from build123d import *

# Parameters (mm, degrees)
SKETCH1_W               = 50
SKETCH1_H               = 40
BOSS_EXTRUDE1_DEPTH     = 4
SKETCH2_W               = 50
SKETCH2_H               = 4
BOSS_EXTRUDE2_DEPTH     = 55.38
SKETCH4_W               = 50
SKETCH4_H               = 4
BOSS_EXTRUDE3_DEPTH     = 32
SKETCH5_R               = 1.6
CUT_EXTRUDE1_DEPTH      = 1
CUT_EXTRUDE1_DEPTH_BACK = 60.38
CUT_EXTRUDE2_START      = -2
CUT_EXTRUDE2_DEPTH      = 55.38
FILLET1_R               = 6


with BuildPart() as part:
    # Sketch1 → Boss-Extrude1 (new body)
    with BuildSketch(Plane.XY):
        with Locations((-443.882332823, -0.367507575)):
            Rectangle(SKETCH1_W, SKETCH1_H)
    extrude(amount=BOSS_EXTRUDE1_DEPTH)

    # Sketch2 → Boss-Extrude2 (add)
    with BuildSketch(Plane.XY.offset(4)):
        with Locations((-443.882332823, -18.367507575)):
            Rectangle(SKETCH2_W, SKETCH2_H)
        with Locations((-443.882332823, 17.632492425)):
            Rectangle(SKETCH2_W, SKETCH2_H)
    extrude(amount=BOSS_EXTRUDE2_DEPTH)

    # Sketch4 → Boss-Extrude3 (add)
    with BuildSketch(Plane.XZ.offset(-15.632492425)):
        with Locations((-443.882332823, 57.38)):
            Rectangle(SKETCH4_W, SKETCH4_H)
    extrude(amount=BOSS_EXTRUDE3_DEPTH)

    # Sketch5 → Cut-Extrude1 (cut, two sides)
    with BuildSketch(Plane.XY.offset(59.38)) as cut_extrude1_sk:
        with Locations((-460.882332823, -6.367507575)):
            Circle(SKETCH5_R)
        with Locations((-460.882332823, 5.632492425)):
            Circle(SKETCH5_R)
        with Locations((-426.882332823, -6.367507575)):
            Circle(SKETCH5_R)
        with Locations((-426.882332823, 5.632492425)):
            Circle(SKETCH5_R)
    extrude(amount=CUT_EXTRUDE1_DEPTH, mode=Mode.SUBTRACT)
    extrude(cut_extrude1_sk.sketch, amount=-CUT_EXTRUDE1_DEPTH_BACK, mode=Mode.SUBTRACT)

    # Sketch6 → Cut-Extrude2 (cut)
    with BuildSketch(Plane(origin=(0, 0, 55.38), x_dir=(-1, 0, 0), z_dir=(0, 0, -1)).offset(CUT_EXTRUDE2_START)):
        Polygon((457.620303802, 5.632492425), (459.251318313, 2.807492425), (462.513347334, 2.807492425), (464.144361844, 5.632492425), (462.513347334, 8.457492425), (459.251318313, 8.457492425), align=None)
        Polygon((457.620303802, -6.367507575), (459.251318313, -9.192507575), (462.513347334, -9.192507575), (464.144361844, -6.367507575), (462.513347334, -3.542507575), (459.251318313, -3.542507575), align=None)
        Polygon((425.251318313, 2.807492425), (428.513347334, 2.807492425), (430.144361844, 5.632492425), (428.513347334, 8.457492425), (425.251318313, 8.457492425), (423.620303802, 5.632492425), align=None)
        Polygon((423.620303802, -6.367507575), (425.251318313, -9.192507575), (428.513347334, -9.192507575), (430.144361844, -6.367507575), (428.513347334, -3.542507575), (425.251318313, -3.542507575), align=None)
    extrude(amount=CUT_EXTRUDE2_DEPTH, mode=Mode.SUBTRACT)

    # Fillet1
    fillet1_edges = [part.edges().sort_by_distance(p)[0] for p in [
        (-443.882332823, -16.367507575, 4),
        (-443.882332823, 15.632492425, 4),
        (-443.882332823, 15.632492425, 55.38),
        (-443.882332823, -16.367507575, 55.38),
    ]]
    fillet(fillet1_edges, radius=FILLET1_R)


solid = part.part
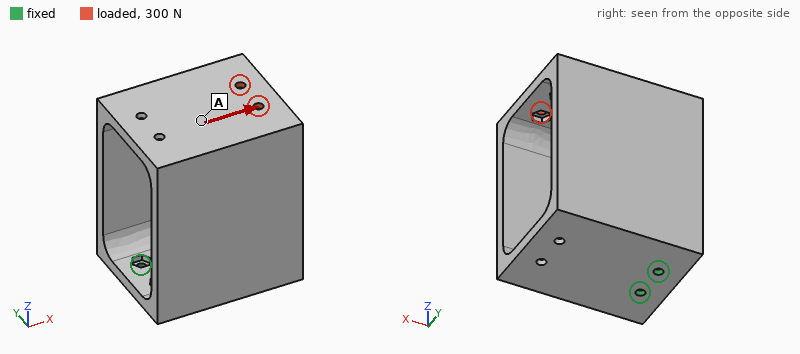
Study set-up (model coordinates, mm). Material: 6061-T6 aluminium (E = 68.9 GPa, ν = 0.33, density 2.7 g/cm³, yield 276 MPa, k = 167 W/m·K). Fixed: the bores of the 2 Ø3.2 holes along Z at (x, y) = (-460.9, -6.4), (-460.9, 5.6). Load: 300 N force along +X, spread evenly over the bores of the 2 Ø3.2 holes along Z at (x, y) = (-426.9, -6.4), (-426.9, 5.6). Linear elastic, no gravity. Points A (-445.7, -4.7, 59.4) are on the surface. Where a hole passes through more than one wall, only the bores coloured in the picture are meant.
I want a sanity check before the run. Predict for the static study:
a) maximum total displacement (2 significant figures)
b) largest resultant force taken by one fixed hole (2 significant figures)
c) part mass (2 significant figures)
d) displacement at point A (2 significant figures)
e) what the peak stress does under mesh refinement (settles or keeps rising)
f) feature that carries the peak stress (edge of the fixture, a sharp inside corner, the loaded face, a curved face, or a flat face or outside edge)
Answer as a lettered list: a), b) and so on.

a) 1.0 mm
b) 280 N
c) 100 g
d) 0.86 mm
e) keeps rising
f) edge of the fixture
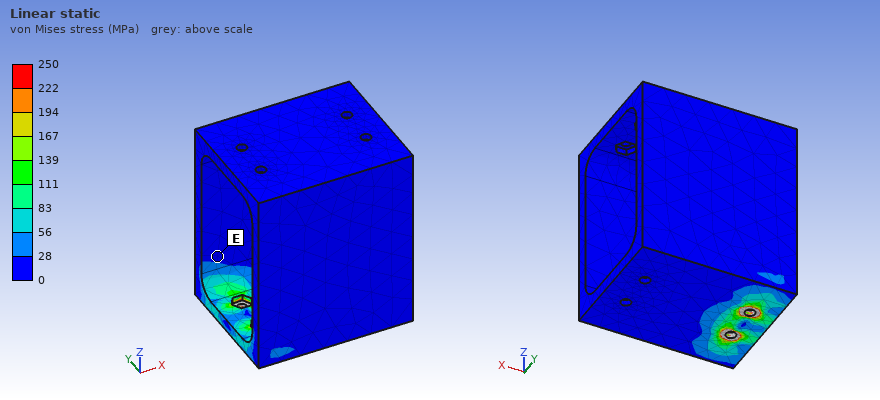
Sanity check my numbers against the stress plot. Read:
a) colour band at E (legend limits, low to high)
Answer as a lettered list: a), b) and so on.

a) 0 to 28 MPa
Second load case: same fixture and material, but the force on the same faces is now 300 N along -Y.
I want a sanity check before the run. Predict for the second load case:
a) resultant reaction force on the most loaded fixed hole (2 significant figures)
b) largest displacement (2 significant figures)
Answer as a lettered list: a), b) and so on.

a) 1.3 kN
b) 0.40 mm
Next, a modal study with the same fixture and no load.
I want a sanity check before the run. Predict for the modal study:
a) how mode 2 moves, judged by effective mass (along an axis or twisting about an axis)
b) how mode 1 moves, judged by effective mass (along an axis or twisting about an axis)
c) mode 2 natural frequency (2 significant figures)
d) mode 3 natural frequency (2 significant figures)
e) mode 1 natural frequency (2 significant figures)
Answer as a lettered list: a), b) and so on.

a) along Y
b) along X
c) 650 Hz
d) 2000 Hz
e) 410 Hz
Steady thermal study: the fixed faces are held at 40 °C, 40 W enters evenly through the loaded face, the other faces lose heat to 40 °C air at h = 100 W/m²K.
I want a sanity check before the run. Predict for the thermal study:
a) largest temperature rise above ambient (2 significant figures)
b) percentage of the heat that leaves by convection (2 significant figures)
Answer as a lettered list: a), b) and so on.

a) 48 K
b) 71 %
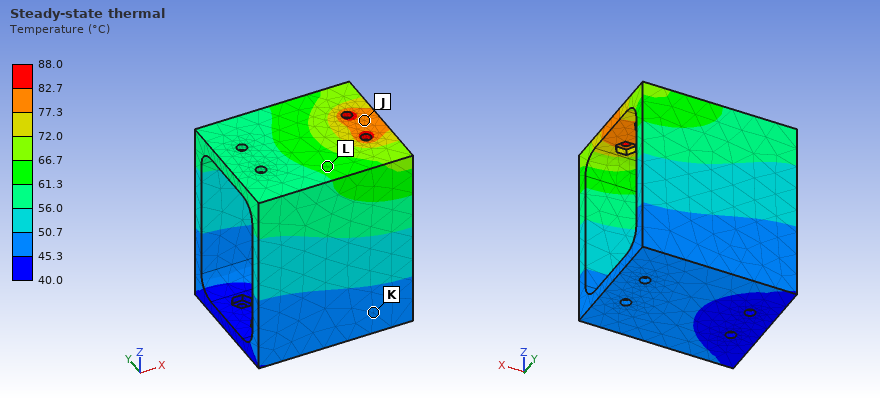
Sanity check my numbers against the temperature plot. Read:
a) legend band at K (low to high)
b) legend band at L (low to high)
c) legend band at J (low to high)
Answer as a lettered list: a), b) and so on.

a) 45.3 to 50.7 °C
b) 61.3 to 66.7 °C
c) 77.3 to 82.7 °C
